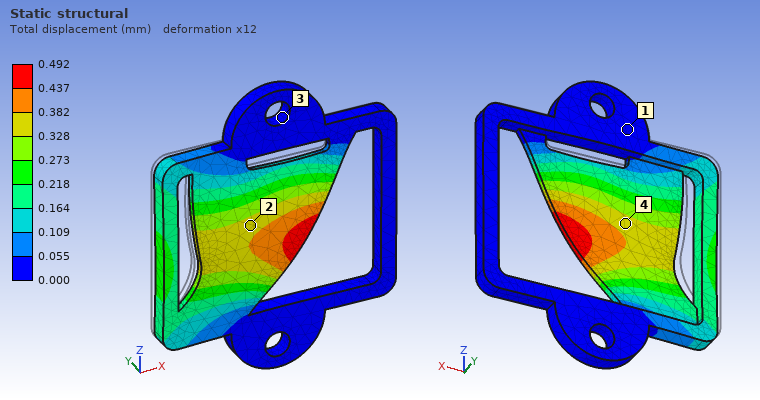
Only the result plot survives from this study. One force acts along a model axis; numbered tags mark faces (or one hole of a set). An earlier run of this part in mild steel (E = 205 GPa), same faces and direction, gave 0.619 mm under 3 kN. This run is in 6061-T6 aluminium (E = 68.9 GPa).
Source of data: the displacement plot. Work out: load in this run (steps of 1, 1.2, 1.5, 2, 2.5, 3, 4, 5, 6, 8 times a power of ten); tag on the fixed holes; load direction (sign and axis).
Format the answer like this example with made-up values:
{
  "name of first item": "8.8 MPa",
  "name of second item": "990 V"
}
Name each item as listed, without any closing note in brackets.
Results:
{
  "load in this run": "800 N",
  "tag on the fixed holes": "3",
  "load direction": "-Y"
}
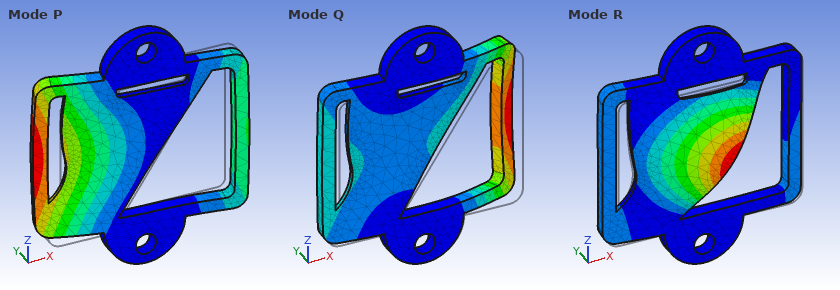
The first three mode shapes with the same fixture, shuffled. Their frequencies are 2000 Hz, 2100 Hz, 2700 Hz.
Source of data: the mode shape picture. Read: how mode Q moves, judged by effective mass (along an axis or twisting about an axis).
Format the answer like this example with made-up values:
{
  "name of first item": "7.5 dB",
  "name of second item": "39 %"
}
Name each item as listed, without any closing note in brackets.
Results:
{
  "how mode Q moves, judged by effective mass": "along Y"
}
